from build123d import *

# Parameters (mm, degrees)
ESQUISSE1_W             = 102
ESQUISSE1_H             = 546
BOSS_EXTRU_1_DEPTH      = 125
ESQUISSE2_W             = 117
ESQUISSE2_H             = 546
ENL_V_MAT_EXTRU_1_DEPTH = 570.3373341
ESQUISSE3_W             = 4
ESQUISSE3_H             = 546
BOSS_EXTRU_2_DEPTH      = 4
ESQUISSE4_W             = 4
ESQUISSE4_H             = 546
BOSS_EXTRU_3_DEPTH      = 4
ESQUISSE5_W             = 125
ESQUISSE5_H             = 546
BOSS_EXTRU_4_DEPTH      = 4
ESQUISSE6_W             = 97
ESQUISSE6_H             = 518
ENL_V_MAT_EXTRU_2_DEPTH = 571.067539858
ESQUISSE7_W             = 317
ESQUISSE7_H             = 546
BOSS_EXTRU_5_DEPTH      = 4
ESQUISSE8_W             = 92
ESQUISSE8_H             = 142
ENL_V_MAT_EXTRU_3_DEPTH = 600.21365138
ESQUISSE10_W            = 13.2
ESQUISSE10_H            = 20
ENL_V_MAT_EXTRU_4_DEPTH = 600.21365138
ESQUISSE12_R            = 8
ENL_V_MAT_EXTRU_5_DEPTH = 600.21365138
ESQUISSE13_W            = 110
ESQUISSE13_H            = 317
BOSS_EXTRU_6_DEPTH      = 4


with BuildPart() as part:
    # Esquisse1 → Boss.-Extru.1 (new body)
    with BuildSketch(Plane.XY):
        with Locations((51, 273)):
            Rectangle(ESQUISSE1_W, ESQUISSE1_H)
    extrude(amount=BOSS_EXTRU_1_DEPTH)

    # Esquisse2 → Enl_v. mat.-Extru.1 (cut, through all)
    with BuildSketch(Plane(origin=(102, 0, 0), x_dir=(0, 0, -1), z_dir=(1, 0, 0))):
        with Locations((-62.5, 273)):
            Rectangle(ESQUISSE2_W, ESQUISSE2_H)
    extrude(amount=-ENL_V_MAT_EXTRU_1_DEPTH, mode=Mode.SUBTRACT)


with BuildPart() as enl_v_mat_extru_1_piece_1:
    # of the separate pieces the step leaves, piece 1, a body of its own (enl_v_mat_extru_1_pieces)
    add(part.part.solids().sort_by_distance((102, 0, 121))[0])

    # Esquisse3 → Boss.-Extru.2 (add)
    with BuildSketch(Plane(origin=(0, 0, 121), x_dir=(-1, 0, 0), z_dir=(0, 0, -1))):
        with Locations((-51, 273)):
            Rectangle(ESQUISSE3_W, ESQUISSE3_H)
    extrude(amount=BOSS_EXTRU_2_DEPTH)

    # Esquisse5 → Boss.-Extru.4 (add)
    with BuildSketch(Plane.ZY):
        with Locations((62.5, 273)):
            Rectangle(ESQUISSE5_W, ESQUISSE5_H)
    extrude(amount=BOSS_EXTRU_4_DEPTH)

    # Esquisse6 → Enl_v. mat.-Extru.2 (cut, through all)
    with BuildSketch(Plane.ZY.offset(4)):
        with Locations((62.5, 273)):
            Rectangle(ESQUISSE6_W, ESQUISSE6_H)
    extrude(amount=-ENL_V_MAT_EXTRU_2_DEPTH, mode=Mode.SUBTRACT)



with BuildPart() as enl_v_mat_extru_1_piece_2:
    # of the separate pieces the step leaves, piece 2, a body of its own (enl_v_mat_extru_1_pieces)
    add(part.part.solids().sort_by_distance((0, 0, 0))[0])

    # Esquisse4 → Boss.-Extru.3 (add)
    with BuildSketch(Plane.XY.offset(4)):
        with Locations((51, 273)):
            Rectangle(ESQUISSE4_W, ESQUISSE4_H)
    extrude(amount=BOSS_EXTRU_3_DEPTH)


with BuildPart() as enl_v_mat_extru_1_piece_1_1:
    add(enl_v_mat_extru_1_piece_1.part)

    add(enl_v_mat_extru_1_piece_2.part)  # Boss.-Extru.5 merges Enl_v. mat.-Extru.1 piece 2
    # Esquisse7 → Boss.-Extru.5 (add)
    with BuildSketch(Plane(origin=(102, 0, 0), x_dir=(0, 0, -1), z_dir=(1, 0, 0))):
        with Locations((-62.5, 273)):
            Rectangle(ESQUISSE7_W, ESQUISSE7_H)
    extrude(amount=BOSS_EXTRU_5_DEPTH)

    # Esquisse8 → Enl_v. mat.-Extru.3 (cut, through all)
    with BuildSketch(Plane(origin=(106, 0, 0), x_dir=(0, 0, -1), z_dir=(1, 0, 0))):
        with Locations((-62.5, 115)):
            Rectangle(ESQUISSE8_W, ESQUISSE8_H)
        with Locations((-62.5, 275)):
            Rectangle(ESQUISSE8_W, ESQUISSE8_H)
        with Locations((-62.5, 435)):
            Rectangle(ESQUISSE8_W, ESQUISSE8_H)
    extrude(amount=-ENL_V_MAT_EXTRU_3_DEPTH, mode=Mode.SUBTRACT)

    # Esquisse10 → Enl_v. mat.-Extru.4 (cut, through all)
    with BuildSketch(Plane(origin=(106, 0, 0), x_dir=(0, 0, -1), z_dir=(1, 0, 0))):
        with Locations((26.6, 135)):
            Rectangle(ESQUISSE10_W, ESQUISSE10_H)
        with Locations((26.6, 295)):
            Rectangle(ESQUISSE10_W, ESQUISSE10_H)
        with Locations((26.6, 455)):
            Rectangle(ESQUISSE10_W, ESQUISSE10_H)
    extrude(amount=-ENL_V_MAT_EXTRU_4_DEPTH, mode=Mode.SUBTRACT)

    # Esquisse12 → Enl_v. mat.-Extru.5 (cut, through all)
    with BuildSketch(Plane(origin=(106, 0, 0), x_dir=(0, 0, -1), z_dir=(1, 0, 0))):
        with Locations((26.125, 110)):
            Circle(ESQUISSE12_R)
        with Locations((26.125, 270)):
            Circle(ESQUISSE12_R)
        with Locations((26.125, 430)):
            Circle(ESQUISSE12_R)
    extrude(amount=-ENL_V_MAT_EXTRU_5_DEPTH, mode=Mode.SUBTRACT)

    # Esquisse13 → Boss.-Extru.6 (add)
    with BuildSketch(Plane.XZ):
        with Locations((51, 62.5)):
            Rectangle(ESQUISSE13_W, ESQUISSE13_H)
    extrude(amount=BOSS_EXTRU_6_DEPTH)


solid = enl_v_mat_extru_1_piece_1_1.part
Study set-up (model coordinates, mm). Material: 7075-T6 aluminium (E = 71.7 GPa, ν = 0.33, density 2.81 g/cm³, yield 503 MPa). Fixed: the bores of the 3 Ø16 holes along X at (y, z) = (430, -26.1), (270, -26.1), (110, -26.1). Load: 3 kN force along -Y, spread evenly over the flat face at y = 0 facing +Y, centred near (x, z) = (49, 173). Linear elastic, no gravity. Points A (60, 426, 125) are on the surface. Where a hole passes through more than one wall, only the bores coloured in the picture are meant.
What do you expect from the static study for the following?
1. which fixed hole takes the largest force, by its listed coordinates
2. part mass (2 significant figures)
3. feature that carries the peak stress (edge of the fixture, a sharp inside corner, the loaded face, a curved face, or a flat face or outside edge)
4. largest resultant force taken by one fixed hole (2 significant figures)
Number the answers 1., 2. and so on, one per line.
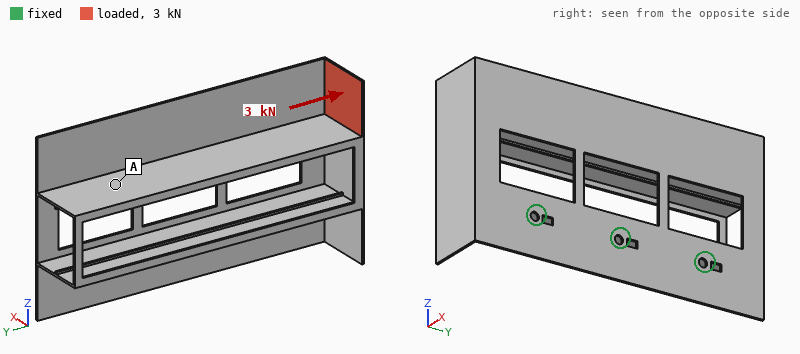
1. (110, -26.1)
2. 3.4 kg
3. a flat face or outside edge
4. 2.4 kN
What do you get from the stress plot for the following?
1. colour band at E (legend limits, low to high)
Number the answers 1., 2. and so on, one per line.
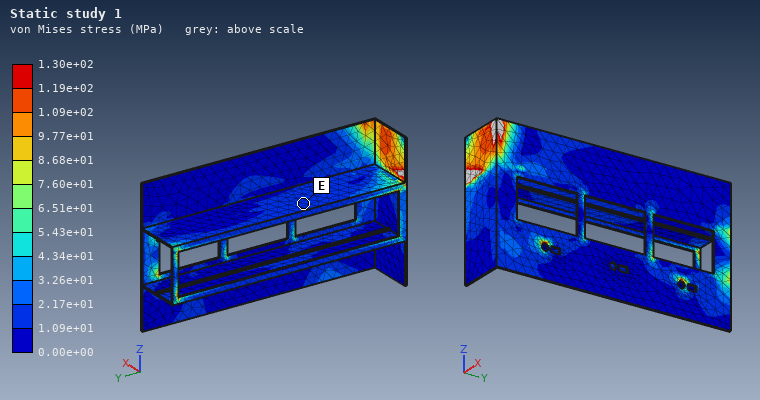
1. 1.09e+01 to 2.17e+01 MPa
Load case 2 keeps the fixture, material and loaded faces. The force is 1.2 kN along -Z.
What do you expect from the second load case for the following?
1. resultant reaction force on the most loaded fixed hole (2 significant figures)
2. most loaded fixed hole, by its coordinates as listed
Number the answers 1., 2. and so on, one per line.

1. 1.7 kN
2. (110, -26.1)
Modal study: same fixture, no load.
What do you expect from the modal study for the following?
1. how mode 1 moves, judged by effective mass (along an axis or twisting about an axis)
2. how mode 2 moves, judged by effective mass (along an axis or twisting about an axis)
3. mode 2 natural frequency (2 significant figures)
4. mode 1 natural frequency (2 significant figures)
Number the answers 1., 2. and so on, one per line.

1. along X
2. twisting about Z
3. 86 Hz
4. 40 Hz
